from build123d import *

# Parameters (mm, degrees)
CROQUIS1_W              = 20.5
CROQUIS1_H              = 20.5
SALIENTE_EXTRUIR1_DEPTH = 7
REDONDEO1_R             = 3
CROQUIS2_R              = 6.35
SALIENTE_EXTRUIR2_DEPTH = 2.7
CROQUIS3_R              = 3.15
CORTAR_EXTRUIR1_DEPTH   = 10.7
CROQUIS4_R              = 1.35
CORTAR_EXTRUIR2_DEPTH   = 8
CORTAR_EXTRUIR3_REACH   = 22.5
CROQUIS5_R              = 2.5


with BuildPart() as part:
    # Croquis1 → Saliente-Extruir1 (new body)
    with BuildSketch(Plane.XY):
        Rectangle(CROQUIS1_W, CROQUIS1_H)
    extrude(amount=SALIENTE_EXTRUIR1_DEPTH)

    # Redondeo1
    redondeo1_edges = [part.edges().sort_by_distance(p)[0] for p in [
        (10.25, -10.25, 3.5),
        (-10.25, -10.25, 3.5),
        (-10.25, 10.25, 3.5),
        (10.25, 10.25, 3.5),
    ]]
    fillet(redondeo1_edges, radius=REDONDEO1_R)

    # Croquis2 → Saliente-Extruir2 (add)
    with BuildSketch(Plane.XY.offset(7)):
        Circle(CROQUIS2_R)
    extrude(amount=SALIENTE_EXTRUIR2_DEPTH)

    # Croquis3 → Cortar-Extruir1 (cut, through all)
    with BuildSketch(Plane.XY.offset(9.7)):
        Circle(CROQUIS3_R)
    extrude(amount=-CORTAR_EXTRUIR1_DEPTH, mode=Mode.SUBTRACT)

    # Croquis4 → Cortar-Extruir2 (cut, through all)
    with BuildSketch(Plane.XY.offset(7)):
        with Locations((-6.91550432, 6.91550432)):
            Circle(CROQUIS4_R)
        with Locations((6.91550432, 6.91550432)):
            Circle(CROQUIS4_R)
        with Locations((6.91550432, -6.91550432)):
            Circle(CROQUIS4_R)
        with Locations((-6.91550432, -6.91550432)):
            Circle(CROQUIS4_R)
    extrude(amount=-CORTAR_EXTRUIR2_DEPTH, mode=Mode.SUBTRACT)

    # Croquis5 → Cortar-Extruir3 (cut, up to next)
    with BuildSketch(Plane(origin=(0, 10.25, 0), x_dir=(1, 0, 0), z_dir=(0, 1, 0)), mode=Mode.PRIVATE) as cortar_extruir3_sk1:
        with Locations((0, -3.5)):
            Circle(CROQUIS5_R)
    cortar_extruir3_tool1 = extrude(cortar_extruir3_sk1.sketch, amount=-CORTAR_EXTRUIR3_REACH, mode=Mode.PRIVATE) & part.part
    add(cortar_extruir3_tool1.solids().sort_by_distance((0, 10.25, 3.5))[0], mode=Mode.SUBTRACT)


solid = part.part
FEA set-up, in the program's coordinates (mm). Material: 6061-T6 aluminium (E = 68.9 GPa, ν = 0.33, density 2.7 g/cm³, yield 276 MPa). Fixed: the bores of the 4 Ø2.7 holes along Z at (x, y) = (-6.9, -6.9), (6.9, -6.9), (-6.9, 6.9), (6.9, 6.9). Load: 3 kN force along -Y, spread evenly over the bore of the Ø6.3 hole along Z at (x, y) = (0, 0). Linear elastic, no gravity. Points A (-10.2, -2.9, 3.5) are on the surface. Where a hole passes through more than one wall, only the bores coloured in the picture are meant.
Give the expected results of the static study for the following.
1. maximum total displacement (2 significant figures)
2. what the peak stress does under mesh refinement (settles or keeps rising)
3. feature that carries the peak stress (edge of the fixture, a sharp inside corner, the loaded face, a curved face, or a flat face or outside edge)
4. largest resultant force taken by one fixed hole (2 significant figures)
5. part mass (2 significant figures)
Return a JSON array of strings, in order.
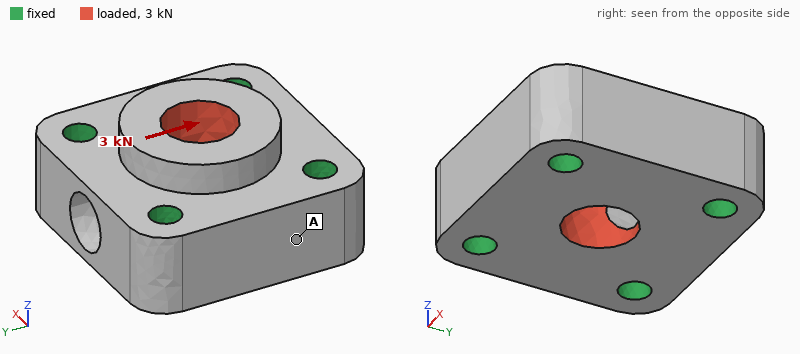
["4.8 µm", "keeps rising", "edge of the fixture", "880 N", "7.1 g"]
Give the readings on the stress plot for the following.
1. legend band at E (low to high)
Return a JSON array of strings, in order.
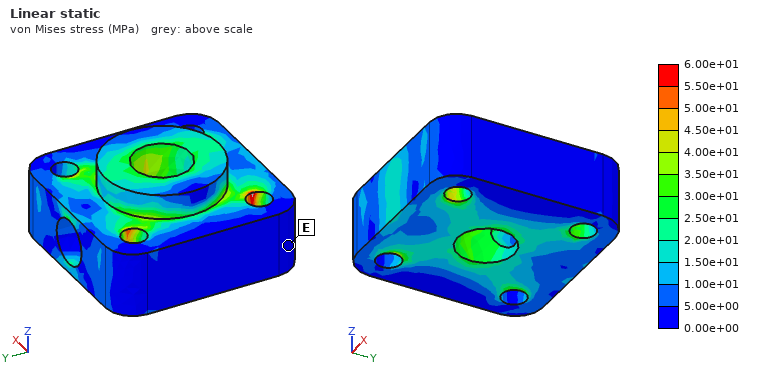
["0.00e+00 to 5.00e+00 MPa"]
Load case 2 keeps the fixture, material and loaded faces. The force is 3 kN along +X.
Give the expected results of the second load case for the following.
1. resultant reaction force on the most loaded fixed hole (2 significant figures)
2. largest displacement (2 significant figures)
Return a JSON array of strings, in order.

["940 N", "5.1 µm"]
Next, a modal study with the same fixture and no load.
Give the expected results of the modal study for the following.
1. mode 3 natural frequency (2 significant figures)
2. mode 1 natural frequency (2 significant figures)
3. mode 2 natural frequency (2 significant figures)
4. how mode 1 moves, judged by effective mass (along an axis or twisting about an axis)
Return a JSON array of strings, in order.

["95 kHz", "84 kHz", "92 kHz", "along Z"]
